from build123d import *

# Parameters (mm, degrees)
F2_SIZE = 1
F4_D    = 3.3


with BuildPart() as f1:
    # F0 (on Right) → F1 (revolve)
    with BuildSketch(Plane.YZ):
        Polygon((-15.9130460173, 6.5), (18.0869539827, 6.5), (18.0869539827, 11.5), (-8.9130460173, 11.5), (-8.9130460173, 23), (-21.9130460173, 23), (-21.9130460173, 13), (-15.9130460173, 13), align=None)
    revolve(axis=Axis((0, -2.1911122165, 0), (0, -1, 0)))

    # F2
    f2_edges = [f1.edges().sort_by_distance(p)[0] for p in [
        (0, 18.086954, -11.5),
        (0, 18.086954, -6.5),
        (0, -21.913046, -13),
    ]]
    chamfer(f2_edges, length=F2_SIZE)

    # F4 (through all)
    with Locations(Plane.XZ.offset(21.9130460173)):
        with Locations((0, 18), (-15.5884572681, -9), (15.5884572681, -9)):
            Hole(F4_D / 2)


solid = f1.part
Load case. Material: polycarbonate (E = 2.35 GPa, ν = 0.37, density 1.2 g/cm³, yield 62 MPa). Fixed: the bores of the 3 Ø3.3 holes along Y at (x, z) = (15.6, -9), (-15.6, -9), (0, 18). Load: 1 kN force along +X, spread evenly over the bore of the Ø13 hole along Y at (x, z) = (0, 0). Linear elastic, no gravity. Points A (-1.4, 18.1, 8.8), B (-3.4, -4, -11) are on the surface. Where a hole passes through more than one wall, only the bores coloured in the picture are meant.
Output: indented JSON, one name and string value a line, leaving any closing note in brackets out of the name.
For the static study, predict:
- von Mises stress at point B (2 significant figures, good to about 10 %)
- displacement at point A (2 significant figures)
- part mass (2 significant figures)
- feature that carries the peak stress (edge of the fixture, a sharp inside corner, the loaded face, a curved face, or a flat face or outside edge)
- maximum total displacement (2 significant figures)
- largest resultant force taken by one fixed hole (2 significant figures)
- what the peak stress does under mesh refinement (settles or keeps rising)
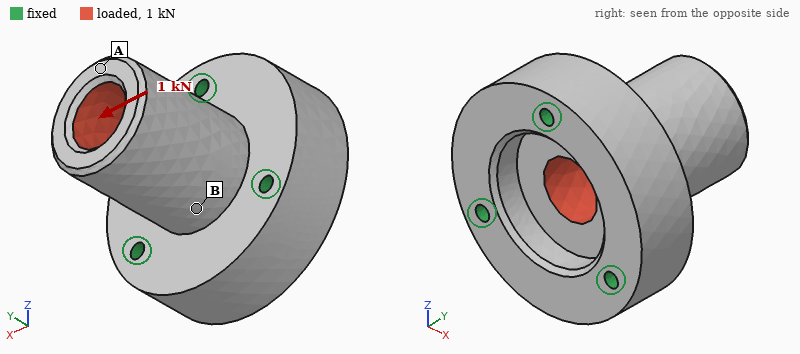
{
  "von Mises stress at point B": "5.2 MPa",
  "displacement at point A": "0.25 mm",
  "part mass": "30 g",
  "feature that carries the peak stress": "edge of the fixture",
  "maximum total displacement": "0.27 mm",
  "largest resultant force taken by one fixed hole": "550 N",
  "what the peak stress does under mesh refinement": "keeps rising"
}
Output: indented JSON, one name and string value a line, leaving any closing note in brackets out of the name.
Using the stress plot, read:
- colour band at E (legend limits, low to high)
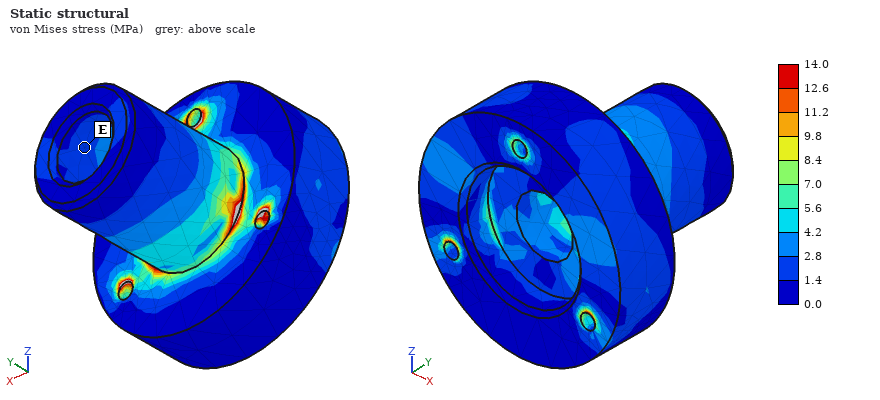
{
  "colour band at E": "1.4 to 2.8 MPa"
}
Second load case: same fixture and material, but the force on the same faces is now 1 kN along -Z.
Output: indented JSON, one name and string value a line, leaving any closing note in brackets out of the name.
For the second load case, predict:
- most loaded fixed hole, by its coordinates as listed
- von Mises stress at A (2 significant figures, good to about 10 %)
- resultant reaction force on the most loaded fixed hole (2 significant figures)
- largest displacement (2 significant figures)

{
  "most loaded fixed hole, by its coordinates as listed": "(0, 18)",
  "von Mises stress at A": "1.4 MPa",
  "resultant reaction force on the most loaded fixed hole": "610 N",
  "largest displacement": "0.27 mm"
}
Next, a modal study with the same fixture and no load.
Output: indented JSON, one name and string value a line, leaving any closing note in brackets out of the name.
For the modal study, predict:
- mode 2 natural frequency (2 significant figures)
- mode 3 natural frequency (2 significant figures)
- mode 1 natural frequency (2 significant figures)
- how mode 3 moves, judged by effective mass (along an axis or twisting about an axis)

{
  "mode 2 natural frequency": "3300 Hz",
  "mode 3 natural frequency": "6400 Hz",
  "mode 1 natural frequency": "3300 Hz",
  "how mode 3 moves, judged by effective mass": "along Y"
}
